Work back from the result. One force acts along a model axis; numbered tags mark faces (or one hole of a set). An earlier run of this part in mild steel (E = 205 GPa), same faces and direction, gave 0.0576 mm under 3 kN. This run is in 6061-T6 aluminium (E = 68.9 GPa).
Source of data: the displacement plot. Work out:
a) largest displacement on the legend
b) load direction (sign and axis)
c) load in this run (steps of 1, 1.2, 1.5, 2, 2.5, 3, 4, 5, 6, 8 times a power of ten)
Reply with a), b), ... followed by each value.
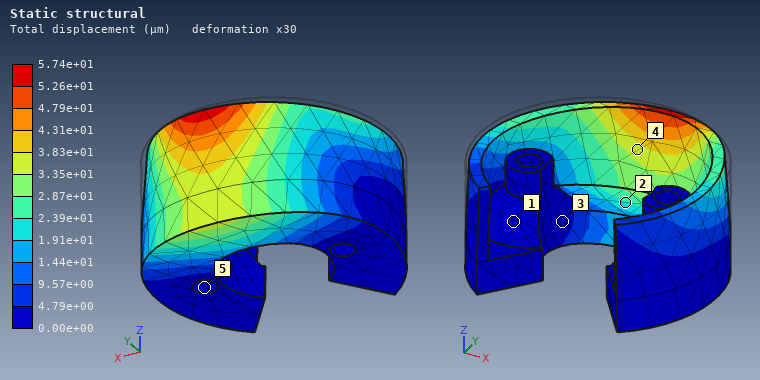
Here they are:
a) 5.74e+01 µm
b) -Z
c) 1 kN
